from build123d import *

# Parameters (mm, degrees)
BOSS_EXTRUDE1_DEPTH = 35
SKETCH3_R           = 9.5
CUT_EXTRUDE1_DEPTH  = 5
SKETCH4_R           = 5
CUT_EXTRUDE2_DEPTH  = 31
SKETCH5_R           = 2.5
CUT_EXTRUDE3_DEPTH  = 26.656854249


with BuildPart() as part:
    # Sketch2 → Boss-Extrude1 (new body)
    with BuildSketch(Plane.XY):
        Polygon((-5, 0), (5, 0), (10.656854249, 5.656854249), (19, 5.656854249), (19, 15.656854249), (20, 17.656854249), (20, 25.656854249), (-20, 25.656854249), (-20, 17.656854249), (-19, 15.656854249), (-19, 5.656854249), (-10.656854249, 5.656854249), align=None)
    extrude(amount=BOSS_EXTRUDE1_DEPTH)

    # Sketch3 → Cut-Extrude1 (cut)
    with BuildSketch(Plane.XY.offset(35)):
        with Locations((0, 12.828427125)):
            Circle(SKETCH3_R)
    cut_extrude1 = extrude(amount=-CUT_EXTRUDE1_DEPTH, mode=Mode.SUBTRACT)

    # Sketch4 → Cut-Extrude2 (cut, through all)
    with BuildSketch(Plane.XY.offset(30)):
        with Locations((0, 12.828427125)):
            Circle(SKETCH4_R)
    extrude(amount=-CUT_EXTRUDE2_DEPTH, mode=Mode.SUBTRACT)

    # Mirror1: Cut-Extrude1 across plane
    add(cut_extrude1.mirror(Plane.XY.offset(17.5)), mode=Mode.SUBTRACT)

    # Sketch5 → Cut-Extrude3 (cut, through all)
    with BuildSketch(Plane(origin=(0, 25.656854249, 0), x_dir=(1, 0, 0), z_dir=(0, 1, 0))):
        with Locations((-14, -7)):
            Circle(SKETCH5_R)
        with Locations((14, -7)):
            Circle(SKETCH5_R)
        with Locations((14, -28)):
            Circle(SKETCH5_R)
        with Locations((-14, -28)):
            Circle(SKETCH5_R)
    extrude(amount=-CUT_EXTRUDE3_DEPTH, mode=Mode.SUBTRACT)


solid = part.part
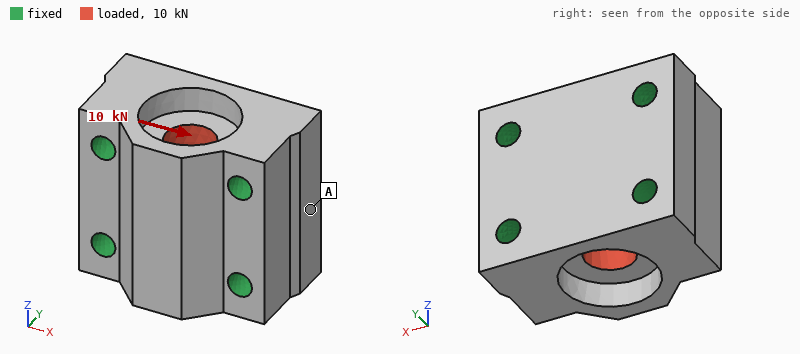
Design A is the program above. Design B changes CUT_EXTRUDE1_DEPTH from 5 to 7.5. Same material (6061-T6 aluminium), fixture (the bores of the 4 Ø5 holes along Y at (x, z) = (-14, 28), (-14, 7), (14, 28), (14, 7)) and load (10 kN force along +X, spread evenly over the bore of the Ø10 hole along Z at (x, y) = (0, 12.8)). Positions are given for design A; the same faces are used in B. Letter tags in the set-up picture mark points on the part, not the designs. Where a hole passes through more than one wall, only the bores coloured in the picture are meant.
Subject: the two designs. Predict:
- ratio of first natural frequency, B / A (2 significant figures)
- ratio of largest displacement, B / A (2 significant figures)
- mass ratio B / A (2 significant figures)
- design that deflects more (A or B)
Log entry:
0.99
1.3
0.96
B
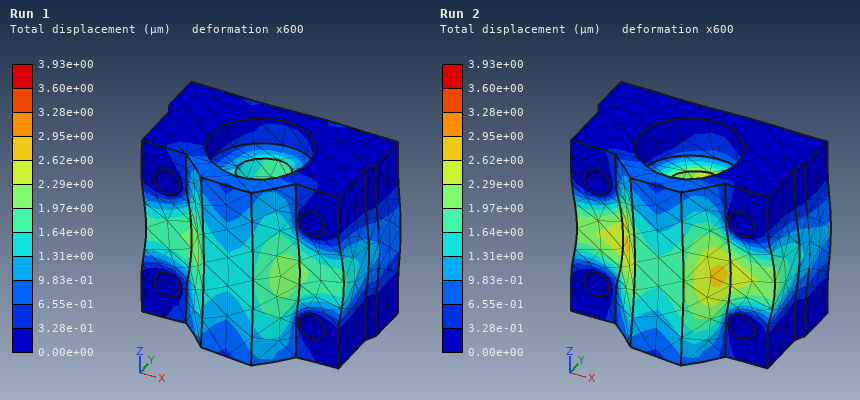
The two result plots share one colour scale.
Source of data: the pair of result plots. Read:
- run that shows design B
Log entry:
Run 2
